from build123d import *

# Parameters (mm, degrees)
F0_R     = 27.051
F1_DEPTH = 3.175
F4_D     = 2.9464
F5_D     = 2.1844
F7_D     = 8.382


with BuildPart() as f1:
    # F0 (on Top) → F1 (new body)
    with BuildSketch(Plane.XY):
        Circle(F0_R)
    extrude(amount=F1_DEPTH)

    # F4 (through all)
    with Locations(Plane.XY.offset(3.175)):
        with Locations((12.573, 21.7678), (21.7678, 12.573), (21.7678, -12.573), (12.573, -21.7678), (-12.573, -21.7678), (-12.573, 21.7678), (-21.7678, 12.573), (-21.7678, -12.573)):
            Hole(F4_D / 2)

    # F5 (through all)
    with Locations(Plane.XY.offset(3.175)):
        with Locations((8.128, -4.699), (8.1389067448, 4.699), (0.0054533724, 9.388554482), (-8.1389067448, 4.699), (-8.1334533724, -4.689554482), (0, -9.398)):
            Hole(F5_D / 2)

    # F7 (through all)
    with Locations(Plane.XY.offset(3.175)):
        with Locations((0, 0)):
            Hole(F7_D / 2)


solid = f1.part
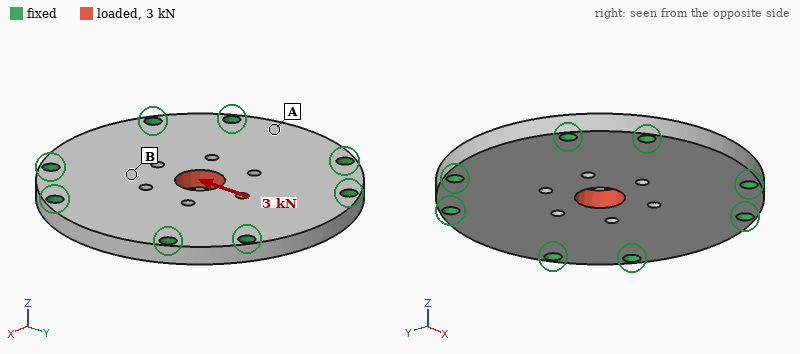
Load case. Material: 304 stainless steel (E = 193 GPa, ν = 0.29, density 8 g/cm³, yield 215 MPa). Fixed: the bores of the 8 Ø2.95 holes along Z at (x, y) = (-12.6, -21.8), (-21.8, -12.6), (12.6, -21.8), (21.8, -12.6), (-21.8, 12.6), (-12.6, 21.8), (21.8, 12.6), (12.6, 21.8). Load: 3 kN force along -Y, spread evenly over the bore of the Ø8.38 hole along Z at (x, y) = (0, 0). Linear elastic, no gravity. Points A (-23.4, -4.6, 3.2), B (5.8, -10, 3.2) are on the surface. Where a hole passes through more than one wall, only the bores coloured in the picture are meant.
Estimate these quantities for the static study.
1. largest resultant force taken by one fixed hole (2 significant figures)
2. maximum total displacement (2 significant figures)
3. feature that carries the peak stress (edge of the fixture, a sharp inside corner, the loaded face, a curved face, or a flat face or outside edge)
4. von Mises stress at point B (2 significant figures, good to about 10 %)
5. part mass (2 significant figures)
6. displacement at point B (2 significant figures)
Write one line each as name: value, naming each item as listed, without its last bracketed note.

largest resultant force taken by one fixed hole: 560 N
maximum total displacement: 2.9 µm
feature that carries the peak stress: a curved face
von Mises stress at point B: 23 MPa
part mass: 55 g
displacement at point B: 1.5 µm
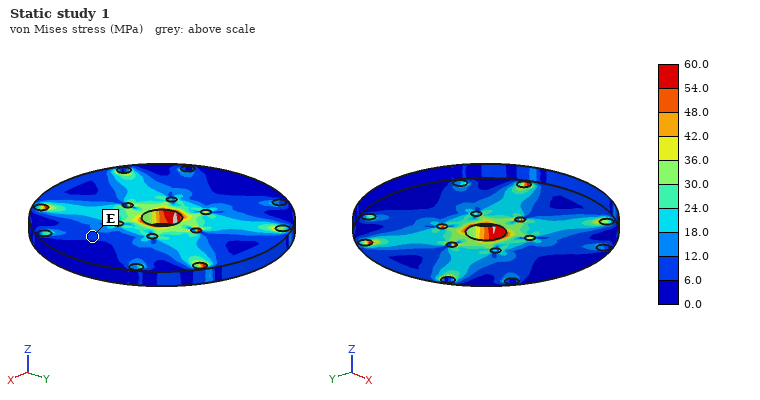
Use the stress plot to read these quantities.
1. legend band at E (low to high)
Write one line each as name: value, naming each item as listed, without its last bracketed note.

legend band at E: 6.0 to 12.0 MPa
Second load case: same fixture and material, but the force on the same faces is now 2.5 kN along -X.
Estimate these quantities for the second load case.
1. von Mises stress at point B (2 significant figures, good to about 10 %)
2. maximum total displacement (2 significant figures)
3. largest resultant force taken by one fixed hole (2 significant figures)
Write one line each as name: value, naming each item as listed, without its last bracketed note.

von Mises stress at point B: 14 MPa
maximum total displacement: 2.4 µm
largest resultant force taken by one fixed hole: 460 N
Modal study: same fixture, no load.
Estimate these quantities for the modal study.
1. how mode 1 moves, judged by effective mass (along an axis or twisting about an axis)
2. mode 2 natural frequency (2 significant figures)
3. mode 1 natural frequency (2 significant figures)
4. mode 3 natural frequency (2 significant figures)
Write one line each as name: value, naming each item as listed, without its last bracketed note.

how mode 1 moves, judged by effective mass: along Z
mode 2 natural frequency: 20 kHz
mode 1 natural frequency: 10 kHz
mode 3 natural frequency: 20 kHz
